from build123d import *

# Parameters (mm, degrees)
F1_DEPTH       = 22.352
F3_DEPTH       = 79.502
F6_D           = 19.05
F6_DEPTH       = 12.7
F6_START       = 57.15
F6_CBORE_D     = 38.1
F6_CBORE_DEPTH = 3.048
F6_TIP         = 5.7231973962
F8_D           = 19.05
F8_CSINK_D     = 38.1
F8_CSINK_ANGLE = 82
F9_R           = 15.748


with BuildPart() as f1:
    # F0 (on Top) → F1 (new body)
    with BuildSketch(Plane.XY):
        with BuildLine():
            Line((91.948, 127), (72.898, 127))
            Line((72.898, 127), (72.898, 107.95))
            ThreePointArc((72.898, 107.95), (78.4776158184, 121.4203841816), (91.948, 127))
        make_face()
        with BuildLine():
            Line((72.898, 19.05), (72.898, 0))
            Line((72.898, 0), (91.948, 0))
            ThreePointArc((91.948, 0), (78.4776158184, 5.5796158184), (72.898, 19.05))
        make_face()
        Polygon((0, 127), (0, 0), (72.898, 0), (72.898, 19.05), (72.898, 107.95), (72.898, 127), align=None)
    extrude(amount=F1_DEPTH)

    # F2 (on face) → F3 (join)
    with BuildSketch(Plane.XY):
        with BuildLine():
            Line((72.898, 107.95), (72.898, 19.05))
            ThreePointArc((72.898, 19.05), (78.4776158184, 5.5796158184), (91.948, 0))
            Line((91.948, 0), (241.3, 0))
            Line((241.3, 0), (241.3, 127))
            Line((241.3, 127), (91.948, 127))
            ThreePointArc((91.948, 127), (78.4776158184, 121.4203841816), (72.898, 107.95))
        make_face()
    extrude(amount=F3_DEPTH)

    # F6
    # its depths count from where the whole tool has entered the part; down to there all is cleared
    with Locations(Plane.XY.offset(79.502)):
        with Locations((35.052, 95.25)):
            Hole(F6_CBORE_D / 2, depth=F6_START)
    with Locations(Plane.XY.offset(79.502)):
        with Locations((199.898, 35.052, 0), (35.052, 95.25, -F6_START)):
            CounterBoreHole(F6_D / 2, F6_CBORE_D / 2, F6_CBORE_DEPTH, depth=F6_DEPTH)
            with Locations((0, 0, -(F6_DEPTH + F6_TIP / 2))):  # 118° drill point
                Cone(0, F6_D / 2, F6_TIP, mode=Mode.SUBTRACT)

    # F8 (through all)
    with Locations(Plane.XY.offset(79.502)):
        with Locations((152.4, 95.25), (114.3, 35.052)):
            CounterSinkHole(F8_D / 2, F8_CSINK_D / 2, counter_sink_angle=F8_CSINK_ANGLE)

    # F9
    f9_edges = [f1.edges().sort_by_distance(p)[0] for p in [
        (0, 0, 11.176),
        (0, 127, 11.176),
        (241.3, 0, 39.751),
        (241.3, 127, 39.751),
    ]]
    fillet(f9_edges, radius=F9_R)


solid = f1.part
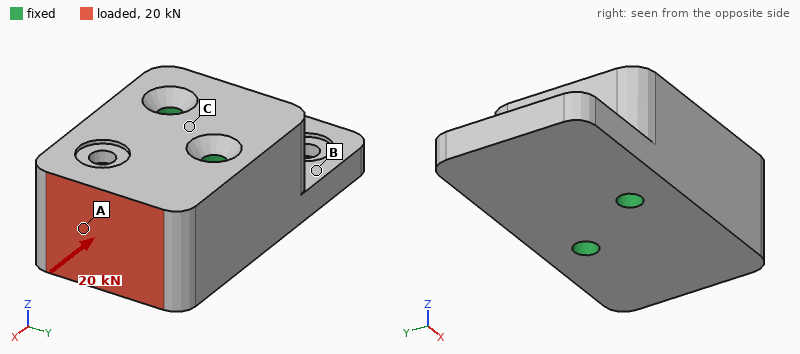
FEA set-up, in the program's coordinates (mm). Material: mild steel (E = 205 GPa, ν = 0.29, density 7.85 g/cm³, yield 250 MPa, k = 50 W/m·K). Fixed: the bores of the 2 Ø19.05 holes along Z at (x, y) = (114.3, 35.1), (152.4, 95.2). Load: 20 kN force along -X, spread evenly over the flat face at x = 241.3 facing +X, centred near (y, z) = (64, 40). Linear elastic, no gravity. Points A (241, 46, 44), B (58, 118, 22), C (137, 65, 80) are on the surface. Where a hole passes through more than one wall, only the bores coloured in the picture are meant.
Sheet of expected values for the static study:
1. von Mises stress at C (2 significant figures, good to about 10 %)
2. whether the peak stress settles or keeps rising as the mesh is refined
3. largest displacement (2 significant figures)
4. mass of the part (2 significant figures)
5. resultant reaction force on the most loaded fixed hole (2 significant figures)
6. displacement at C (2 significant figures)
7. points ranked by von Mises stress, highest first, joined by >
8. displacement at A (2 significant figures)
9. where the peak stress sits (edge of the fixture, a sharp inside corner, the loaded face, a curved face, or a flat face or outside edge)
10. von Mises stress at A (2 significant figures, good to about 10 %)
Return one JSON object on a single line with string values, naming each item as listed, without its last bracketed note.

{"von Mises stress at C": "1.2 MPa", "whether the peak stress settles or keeps rising as the mesh is refined": "keeps rising", "largest displacement": "1.8 µm", "mass of the part": "14 kg", "resultant reaction force on the most loaded fixed hole": "10 kN", "displacement at C": "0.29 µm", "points ranked by von Mises stress, highest first, joined by >": "A > C > B", "displacement at A": "1.5 µm", "where the peak stress sits": "edge of the fixture", "von Mises stress at A": "2.4 MPa"}
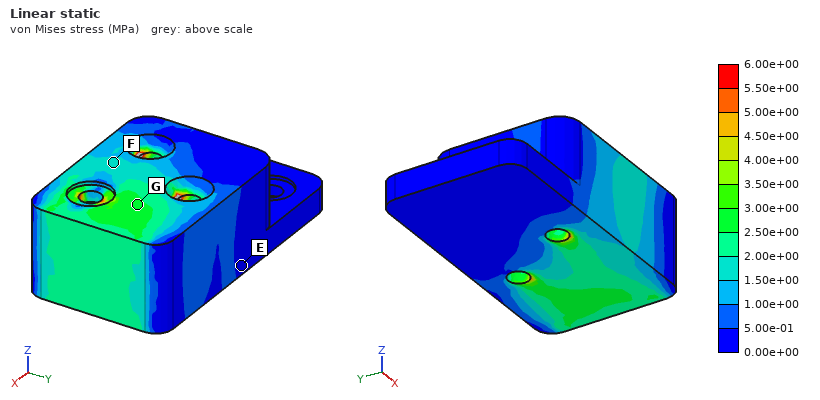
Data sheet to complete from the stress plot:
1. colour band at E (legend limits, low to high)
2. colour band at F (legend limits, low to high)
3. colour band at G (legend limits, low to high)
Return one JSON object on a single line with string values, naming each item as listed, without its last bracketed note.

{"colour band at E": "0.00e+00 to 5.00e-01 MPa", "colour band at F": "1.50e+00 to 2.00e+00 MPa", "colour band at G": "2.50e+00 to 3.00e+00 MPa"}
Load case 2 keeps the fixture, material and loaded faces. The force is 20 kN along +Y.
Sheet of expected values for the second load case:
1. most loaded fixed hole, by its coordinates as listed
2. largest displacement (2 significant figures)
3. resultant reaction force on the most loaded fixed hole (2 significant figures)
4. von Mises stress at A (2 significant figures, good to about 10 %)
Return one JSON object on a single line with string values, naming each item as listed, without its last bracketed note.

{"most loaded fixed hole, by its coordinates as listed": "(152.4, 95.2)", "largest displacement": "7.2 µm", "resultant reaction force on the most loaded fixed hole": "31 kN", "von Mises stress at A": "4.6 MPa"}
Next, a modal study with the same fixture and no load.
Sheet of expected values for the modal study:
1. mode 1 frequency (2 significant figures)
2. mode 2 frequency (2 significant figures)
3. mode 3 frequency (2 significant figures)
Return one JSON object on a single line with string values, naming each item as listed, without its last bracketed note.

{"mode 1 frequency": "2400 Hz", "mode 2 frequency": "4000 Hz", "mode 3 frequency": "4100 Hz"}
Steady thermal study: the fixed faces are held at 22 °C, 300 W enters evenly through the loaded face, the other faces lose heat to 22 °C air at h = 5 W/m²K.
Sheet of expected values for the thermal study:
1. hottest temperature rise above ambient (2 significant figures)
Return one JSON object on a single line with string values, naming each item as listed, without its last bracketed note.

{"hottest temperature rise above ambient": "66 K"}
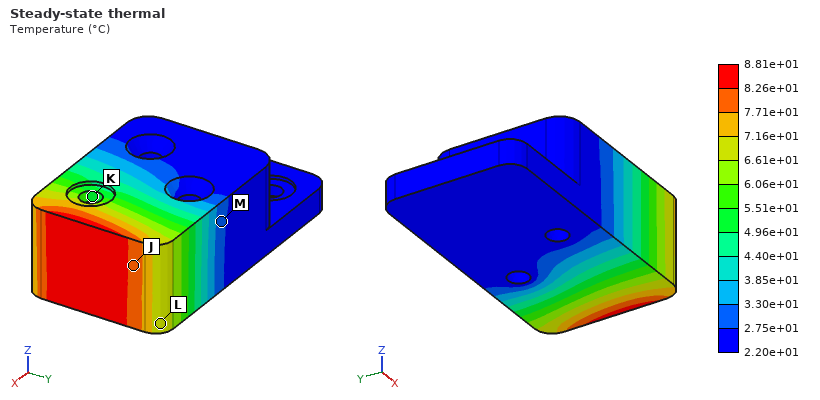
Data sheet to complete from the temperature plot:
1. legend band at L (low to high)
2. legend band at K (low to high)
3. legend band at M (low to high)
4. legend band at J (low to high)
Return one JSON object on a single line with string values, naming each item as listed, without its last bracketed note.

{"legend band at L": "6.61e+01 to 7.16e+01 °C", "legend band at K": "4.96e+01 to 5.51e+01 °C", "legend band at M": "2.75e+01 to 3.30e+01 °C", "legend band at J": "7.71e+01 to 8.26e+01 °C"}
